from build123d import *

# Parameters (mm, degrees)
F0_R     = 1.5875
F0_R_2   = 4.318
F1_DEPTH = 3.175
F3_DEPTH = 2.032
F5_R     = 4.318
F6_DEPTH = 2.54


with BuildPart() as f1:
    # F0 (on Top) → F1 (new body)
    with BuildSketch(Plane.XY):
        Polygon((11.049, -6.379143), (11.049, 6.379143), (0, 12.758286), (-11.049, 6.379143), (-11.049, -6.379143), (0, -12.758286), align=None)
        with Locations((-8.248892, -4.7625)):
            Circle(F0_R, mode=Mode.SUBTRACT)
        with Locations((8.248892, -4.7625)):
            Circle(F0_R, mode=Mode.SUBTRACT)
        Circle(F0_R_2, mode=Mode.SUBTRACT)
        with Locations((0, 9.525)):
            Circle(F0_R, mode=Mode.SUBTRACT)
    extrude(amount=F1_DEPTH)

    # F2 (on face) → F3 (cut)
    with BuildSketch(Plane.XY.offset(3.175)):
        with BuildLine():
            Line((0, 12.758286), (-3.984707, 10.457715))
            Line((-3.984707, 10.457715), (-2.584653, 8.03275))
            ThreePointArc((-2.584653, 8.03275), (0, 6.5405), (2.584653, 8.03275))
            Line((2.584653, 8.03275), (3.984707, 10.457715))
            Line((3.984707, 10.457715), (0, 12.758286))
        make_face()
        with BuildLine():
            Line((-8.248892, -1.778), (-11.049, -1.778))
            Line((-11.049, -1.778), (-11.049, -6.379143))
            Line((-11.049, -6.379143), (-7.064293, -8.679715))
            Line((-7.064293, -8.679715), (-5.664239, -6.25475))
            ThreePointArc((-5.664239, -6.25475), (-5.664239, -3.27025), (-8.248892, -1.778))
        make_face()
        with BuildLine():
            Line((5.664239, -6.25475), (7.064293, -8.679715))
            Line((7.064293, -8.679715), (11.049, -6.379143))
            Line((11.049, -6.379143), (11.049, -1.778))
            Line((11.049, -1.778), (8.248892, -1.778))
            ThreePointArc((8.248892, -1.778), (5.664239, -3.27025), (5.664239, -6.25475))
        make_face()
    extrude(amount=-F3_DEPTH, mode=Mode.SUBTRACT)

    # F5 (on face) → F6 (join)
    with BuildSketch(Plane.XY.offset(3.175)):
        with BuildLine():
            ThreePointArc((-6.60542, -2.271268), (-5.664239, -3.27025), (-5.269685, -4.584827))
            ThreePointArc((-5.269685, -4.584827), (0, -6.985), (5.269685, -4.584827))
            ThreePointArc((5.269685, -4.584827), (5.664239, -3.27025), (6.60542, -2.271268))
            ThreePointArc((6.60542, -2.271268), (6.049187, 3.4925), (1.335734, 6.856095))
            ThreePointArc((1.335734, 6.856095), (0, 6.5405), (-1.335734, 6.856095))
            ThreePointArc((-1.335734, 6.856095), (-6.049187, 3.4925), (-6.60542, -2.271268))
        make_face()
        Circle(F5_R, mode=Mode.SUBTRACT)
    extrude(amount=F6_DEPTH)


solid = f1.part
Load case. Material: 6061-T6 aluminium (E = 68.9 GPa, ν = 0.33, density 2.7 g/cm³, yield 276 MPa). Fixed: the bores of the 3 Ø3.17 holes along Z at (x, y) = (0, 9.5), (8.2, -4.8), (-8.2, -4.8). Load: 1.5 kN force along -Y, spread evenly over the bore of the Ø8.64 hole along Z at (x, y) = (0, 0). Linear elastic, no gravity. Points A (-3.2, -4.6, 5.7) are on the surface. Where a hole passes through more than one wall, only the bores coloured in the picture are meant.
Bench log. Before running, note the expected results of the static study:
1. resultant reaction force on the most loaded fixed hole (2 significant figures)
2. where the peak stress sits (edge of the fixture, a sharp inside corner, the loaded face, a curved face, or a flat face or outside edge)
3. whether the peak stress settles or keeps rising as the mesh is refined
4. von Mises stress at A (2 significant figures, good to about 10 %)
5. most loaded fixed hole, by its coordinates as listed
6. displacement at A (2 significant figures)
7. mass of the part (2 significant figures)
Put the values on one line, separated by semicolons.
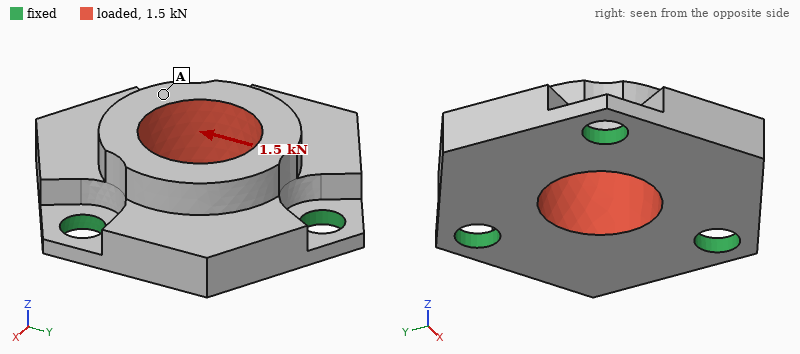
600 N; edge of the fixture; keeps rising; 22 MPa; (0, 9.5); 10 µm; 3.2 g
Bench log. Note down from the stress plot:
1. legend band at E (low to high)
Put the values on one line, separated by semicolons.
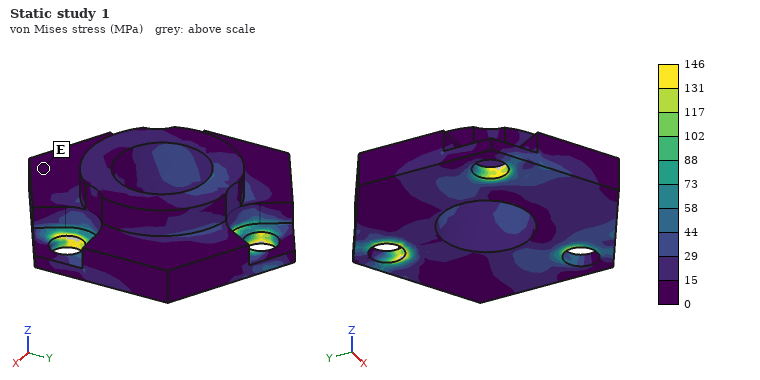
0 to 15 MPa
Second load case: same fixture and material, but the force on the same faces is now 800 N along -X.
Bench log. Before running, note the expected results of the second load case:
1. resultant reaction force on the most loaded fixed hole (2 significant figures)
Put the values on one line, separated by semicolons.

300 N
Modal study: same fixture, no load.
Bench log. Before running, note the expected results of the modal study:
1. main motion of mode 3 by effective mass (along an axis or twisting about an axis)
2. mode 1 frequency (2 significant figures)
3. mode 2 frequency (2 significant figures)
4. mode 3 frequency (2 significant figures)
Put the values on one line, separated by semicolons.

along Z; 27 kHz; 27 kHz; 33 kHz
